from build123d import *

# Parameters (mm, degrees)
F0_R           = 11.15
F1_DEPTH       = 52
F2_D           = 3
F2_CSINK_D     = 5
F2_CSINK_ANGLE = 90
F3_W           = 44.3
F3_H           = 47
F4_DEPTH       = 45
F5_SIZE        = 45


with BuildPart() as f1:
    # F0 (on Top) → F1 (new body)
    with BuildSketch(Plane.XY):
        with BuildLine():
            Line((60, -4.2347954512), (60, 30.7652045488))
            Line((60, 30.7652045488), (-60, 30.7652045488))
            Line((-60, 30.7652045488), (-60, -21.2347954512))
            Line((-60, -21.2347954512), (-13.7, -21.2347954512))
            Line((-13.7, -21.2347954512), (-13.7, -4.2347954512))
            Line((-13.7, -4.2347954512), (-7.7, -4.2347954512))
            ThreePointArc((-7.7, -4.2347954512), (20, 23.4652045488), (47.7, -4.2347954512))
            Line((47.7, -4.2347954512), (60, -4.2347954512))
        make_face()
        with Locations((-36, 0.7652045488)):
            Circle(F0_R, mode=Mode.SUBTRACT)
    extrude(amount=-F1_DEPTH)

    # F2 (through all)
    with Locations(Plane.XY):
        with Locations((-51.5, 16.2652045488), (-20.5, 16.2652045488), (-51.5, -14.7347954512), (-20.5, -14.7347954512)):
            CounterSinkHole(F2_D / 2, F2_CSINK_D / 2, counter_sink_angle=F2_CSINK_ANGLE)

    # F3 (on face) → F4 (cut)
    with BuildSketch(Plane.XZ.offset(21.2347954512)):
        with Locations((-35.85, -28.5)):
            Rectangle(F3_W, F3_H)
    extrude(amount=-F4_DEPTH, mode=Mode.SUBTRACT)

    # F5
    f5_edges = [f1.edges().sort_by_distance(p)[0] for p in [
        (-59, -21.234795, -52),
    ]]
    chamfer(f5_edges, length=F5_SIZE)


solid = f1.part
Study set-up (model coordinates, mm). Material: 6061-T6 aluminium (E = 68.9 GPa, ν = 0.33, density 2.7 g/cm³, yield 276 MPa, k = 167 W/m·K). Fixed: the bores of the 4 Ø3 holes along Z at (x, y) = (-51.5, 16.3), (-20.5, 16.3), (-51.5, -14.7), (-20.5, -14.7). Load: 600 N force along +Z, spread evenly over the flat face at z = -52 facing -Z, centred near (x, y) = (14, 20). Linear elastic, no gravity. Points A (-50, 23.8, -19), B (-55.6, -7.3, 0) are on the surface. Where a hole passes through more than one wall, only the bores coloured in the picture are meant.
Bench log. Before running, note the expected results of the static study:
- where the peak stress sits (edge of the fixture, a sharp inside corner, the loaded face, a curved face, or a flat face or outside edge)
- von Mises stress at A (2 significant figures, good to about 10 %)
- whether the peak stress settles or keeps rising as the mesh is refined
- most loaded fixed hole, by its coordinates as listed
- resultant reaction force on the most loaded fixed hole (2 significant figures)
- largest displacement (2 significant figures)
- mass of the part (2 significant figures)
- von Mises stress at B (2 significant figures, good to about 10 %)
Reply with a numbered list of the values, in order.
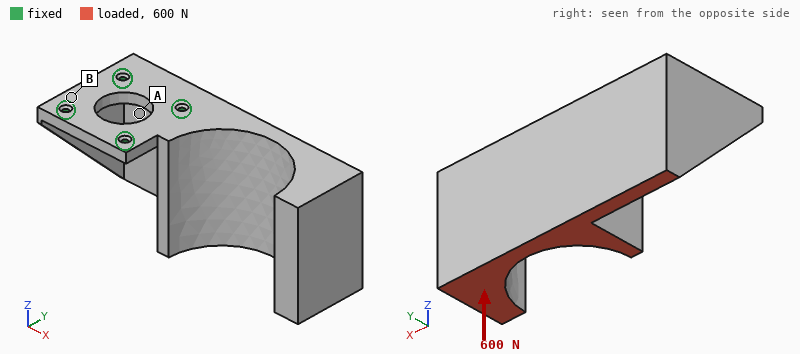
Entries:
1. edge of the fixture
2. 8.9 MPa
3. keeps rising
4. (-20.5, 16.3)
5. 1.2 kN
6. 96 µm
7. 270 g
8. 4.0 MPa
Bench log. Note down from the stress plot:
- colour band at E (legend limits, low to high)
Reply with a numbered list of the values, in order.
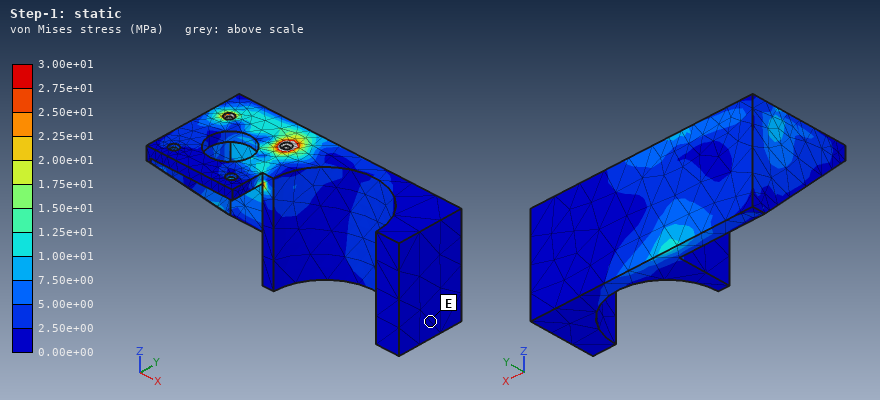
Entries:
1. 0.00e+00 to 2.50e+00 MPa
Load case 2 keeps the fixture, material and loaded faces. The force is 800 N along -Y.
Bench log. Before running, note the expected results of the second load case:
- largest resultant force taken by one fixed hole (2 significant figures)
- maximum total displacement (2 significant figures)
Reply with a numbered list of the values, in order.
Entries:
1. 1.1 kN
2. 0.35 mm
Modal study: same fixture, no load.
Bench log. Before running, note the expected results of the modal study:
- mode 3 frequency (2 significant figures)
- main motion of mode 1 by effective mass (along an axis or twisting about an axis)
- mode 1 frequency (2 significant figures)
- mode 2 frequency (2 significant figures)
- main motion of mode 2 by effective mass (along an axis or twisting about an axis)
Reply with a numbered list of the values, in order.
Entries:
1. 1700 Hz
2. along Y
3. 720 Hz
4. 1000 Hz
5. along Z
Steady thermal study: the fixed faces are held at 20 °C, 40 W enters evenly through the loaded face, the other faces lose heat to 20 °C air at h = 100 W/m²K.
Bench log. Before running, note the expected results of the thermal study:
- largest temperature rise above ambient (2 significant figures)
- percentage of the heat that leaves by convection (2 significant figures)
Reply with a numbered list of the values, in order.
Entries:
1. 17 K
2. 53 %
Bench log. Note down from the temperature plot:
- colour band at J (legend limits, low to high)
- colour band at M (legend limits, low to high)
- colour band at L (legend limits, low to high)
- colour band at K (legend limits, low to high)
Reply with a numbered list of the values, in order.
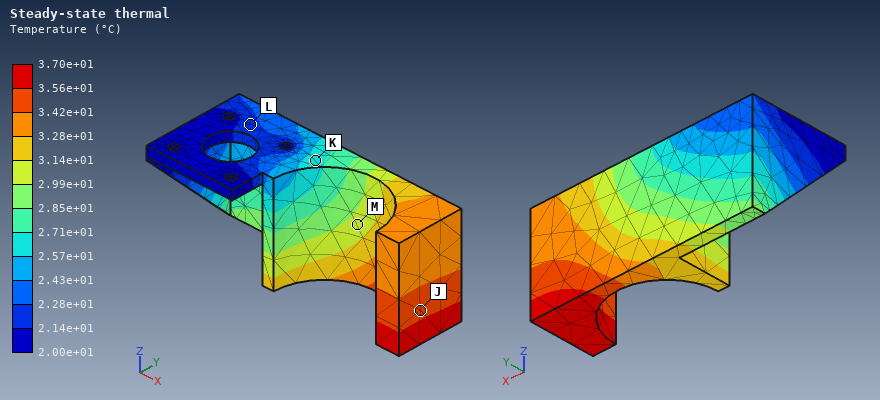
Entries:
1. 3.42e+01 to 3.56e+01 °C
2. 2.99e+01 to 3.14e+01 °C
3. 2.14e+01 to 2.28e+01 °C
4. 2.57e+01 to 2.71e+01 °C
